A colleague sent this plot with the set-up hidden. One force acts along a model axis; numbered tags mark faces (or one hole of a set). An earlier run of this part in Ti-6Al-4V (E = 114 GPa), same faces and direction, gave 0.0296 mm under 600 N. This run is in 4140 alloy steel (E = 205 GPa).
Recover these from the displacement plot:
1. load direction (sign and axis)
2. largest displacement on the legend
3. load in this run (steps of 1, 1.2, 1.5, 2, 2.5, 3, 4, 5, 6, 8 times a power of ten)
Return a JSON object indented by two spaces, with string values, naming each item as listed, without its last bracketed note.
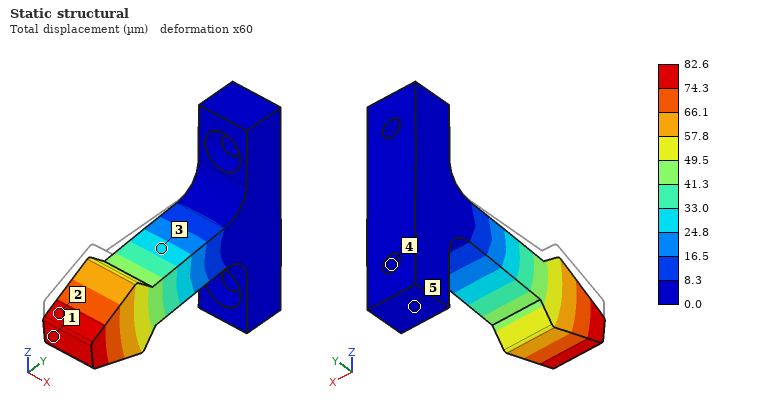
{
  "load direction": "-Z",
  "largest displacement on the legend": "82.6 µm",
  "load in this run": "3 kN"
}
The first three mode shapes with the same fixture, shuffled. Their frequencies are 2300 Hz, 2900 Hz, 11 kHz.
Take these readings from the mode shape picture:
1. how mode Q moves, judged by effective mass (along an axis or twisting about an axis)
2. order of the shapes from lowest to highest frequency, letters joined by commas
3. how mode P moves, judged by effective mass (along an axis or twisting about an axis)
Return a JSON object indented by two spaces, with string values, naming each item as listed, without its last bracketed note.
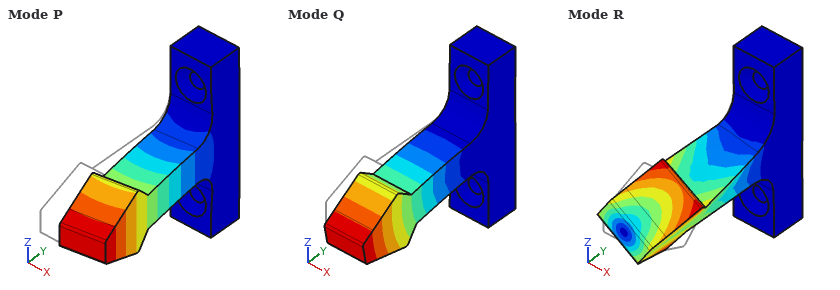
{
  "how mode Q moves, judged by effective mass": "along Z",
  "order of the shapes from lowest to highest frequency, letters joined by commas": "P, Q, R",
  "how mode P moves, judged by effective mass": "along X"
}
